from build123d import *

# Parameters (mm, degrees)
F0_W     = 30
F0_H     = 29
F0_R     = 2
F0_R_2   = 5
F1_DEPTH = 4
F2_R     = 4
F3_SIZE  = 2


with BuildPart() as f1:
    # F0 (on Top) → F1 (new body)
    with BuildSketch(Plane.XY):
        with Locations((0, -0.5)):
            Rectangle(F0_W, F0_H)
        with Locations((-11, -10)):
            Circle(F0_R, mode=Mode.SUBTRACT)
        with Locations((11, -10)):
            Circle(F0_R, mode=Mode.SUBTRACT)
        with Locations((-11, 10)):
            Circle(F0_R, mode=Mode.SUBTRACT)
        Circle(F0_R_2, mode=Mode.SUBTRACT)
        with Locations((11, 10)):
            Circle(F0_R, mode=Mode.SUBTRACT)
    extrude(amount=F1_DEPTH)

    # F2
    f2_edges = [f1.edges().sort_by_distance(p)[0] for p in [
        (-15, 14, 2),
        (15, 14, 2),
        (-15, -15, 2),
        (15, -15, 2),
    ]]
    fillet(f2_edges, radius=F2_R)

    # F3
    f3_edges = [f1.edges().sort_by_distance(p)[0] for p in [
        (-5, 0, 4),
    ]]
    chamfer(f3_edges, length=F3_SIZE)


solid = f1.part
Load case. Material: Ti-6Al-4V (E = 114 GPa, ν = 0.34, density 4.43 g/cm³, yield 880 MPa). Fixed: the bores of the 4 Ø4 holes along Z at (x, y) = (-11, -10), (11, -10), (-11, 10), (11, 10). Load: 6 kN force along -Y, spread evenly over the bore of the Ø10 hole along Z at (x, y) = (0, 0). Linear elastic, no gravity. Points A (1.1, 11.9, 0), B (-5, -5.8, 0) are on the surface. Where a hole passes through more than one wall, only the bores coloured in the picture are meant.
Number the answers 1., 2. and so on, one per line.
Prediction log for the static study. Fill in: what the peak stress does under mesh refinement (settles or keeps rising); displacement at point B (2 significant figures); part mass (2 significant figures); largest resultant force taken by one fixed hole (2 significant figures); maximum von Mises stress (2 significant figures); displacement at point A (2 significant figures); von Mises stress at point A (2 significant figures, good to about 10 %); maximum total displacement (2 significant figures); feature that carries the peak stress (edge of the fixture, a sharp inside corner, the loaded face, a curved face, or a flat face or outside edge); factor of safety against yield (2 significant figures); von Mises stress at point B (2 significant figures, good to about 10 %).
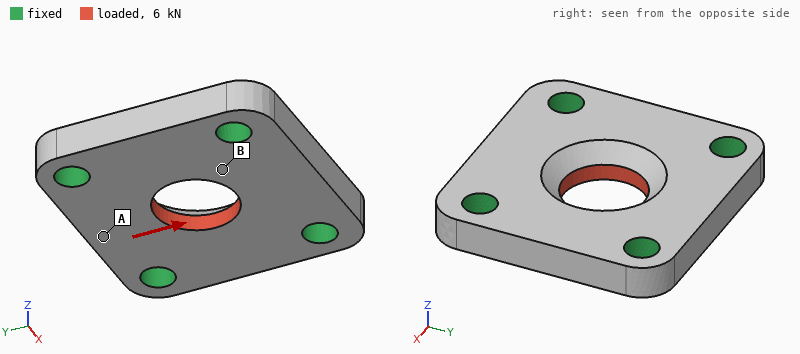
1. settles
2. 4.7 µm
3. 13 g
4. 1.6 kN
5. 190 MPa
6. 6.5 µm
7. 21 MPa
8. 10 µm
9. the loaded face
10. 4.7
11. 81 MPa
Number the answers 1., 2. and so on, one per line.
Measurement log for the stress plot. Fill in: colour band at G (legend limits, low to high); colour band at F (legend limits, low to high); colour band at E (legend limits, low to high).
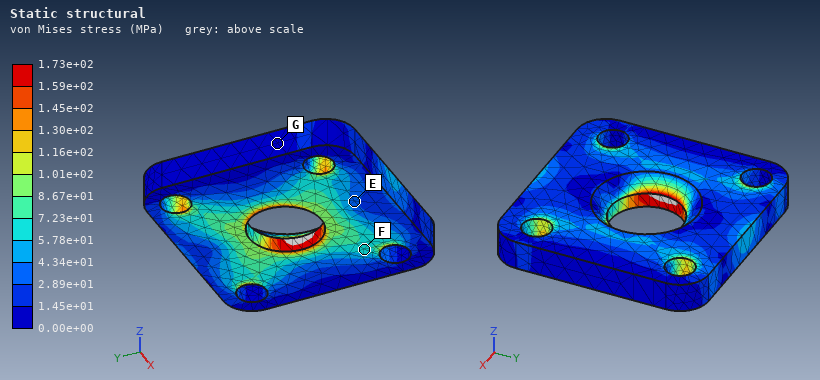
1. 0.00e+00 to 1.45e+01 MPa
2. 5.78e+01 to 7.23e+01 MPa
3. 2.89e+01 to 4.34e+01 MPa
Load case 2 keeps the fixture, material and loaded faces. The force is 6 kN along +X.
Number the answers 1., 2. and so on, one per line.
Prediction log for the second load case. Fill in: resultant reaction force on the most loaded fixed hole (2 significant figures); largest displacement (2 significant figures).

1. 1.6 kN
2. 9.1 µm
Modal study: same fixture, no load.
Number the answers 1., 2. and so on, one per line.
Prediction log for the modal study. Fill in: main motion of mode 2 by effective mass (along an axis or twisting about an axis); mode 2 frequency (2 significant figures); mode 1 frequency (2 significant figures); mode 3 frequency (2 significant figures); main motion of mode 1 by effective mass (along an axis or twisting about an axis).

1. twisting about X
2. 44 kHz
3. 39 kHz
4. 49 kHz
5. along Z
